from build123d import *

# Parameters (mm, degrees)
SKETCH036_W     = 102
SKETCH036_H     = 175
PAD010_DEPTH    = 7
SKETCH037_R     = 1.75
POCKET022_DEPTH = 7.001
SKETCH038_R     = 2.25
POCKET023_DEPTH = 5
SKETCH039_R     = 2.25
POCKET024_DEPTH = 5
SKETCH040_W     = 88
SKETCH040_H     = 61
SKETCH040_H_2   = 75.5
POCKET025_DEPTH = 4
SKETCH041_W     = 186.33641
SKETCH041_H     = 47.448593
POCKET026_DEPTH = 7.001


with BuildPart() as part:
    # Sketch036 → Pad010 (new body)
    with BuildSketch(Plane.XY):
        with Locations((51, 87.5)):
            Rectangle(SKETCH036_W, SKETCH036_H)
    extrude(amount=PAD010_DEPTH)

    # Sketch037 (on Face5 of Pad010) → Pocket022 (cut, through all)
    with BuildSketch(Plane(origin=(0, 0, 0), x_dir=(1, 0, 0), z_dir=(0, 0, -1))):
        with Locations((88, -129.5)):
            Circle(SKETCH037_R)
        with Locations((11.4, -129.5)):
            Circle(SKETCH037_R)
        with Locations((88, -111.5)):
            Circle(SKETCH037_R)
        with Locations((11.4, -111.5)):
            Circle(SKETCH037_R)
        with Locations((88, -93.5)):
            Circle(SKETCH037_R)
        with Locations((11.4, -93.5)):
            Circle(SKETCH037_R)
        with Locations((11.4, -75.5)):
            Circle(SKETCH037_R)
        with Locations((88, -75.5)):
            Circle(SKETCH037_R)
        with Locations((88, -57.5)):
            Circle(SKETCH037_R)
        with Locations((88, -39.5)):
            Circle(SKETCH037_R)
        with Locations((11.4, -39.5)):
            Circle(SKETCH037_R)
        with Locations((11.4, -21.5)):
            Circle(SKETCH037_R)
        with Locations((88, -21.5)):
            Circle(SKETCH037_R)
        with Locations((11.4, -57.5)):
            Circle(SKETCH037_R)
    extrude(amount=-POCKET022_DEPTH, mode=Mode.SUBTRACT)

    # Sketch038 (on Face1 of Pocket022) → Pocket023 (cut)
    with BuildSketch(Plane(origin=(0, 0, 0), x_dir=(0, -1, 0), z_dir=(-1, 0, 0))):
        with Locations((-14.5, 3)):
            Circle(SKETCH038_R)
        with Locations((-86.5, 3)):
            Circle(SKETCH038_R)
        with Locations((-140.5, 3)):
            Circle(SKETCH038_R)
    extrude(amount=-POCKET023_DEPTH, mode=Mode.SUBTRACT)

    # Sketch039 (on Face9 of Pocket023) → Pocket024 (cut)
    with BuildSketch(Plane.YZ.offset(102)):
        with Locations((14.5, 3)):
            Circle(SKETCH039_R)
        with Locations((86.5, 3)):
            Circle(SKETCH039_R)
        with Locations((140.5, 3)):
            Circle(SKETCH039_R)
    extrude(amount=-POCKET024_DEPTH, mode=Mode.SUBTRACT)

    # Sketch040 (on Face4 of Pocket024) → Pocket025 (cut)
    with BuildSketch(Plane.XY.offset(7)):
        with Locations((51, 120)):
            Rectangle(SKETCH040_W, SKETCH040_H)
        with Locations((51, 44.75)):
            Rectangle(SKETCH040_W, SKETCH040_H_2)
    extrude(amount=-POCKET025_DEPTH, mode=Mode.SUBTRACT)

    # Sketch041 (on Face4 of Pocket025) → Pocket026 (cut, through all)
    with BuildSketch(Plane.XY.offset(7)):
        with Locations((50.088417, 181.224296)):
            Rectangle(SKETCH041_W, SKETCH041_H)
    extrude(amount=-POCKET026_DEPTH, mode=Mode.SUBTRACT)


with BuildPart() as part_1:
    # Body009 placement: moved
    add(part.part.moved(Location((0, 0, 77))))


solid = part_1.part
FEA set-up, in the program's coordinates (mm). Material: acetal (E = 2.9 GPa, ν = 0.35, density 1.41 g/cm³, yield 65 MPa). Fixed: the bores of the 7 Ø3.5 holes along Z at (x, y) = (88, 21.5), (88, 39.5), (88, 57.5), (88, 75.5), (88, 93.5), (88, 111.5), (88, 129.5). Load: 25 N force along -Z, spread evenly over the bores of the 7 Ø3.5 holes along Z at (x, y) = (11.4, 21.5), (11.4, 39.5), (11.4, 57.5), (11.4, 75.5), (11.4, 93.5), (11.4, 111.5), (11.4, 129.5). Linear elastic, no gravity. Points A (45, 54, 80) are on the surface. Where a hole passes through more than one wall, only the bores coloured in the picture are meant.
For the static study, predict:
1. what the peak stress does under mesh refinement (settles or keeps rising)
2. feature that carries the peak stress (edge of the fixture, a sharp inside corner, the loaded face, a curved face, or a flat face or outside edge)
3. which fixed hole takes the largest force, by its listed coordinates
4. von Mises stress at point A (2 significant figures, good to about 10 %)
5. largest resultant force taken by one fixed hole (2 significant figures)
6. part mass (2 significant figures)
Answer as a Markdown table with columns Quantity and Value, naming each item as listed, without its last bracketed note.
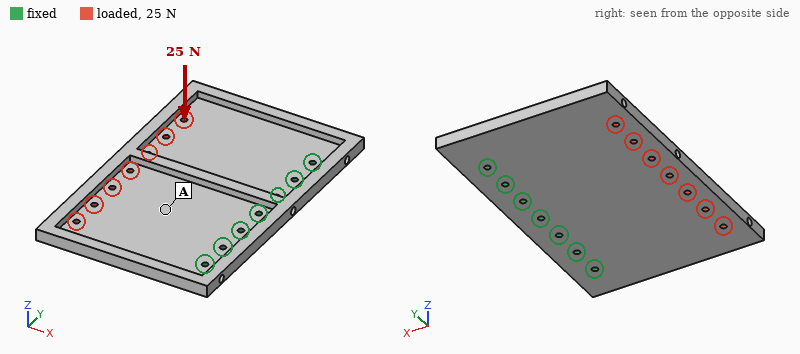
| Quantity | Value |
|---|---|
| what the peak stress does under mesh refinement | keeps rising |
| feature that carries the peak stress | edge of the fixture |
| which fixed hole takes the largest force, by its listed coordinates | (88, 93.5) |
| von Mises stress at point A | 1.0 MPa |
| largest resultant force taken by one fixed hole | 38 N |
| part mass | 90 g |
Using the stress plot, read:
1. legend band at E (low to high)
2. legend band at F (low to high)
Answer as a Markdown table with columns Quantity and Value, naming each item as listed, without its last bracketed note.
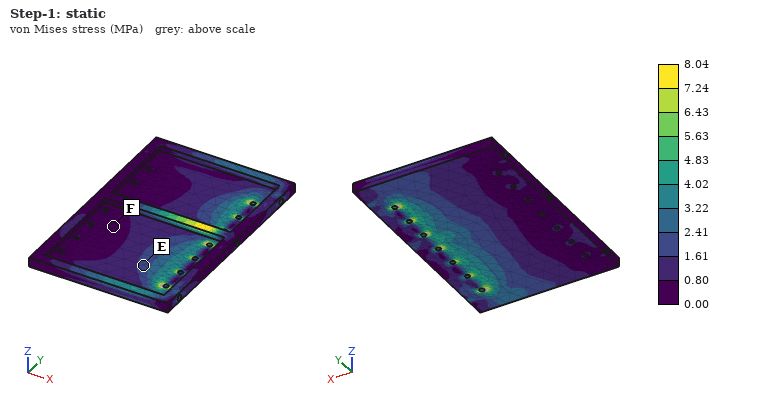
| Quantity | Value |
|---|---|
| legend band at E | 1.61 to 2.41 MPa |
| legend band at F | 0.00 to 0.80 MPa |
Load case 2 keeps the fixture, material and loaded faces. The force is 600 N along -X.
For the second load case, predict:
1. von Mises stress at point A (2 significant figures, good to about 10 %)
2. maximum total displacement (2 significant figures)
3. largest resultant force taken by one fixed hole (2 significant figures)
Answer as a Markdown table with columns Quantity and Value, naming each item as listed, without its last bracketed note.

| Quantity | Value |
|---|---|
| von Mises stress at point A | 1.4 MPa |
| maximum total displacement | 0.19 mm |
| largest resultant force taken by one fixed hole | 110 N |
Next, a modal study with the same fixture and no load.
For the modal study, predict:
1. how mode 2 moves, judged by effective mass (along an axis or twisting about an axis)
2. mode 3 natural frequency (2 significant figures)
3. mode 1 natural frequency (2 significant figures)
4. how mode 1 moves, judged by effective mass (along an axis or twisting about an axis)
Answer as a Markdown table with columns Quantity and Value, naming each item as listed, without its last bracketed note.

| Quantity | Value |
|---|---|
| how mode 2 moves, judged by effective mass | twisting about X |
| mode 3 natural frequency | 380 Hz |
| mode 1 natural frequency | 110 Hz |
| how mode 1 moves, judged by effective mass | along Z |
